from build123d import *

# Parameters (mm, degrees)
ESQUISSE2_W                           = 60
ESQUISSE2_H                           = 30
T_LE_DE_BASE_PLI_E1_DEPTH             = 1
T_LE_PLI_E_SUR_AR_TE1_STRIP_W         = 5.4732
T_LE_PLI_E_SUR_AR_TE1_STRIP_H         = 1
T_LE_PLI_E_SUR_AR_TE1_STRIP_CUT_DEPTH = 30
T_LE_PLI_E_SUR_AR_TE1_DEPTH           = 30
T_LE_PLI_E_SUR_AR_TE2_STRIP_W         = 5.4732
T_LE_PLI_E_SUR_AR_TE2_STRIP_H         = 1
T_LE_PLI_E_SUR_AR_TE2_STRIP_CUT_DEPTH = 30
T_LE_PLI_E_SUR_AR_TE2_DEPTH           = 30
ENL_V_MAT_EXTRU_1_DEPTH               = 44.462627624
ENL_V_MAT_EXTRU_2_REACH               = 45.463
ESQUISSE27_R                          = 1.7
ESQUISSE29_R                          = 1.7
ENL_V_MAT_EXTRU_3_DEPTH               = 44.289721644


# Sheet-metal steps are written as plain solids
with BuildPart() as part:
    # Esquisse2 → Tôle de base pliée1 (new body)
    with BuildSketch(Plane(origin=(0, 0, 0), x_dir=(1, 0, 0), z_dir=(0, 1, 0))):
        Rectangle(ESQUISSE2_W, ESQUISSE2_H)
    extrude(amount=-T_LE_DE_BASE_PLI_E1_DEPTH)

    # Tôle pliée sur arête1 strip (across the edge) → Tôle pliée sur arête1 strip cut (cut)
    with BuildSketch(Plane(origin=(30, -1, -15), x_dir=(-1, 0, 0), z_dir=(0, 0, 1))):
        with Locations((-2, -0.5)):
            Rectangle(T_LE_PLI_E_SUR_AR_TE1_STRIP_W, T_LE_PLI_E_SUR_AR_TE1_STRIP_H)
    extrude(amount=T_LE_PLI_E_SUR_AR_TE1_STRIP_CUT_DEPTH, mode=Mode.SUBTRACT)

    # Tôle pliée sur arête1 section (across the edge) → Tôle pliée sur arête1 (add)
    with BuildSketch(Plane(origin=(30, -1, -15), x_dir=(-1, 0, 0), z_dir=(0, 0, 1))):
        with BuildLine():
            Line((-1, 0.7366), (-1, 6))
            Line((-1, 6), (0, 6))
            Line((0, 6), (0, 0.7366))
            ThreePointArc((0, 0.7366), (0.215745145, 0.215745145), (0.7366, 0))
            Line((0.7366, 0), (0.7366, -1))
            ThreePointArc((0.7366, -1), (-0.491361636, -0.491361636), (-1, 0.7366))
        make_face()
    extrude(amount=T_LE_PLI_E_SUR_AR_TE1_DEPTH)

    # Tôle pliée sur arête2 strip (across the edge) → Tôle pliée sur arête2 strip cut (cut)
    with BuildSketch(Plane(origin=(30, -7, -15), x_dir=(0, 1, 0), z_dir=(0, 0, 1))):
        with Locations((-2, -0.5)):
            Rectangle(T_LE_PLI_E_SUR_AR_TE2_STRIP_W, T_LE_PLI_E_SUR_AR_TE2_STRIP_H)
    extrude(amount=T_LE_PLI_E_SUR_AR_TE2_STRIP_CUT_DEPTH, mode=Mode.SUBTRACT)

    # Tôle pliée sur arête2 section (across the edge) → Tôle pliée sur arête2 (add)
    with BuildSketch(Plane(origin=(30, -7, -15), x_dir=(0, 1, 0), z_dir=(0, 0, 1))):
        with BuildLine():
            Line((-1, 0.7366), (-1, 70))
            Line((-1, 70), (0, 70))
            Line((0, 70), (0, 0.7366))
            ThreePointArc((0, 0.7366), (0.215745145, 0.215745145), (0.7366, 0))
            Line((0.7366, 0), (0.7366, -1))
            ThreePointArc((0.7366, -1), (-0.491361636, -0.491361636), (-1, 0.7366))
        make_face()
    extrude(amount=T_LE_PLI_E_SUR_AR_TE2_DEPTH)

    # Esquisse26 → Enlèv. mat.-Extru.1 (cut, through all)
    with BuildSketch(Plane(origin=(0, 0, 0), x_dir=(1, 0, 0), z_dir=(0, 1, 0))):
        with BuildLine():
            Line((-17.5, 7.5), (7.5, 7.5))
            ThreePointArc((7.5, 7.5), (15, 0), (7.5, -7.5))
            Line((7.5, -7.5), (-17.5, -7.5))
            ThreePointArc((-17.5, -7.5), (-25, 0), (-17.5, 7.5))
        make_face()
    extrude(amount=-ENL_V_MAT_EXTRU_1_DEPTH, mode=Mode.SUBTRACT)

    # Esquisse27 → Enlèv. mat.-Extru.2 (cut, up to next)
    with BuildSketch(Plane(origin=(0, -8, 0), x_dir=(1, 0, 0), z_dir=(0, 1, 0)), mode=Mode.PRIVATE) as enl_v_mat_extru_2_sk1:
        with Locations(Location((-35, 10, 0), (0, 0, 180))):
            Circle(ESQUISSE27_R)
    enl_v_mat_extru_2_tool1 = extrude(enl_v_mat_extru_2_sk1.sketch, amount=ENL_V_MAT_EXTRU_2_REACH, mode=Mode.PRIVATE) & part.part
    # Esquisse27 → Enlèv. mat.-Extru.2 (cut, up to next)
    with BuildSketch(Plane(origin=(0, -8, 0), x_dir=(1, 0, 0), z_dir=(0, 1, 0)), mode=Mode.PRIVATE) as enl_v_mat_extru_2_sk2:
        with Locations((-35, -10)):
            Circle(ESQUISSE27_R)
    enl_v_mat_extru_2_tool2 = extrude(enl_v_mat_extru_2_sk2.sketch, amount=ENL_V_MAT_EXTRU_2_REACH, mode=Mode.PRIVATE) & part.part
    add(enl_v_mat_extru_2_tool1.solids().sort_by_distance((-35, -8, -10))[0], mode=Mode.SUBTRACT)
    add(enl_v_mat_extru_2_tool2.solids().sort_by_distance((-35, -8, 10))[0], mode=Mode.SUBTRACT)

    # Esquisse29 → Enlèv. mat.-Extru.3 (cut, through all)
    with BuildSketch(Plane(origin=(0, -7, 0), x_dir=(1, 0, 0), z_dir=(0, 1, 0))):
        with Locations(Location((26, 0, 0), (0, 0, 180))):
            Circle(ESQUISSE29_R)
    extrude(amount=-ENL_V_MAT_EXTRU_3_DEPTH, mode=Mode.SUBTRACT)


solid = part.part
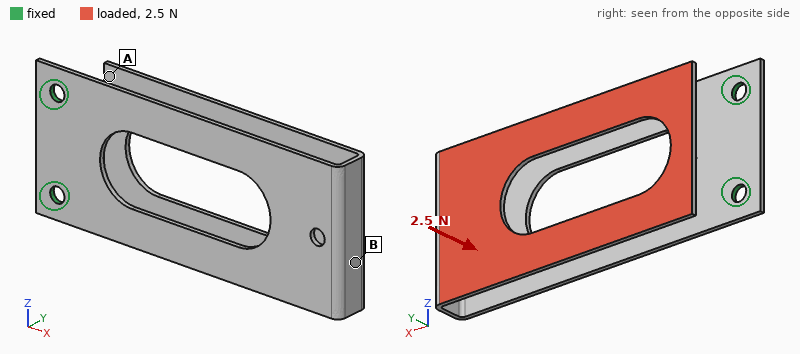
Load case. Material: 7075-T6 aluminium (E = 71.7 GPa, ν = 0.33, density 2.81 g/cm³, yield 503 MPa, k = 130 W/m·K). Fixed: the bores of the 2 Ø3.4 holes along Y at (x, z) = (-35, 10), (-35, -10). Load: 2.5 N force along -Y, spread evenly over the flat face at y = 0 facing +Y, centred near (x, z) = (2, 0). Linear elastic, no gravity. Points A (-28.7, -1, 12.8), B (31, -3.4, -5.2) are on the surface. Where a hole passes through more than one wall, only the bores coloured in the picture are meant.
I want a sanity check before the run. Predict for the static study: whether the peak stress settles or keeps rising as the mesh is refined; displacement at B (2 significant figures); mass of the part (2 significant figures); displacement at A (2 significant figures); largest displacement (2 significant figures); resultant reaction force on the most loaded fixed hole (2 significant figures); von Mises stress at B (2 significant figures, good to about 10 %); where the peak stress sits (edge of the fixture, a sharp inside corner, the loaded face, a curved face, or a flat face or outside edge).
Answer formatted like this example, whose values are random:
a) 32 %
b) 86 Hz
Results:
a) keeps rising
b) 0.62 mm
c) 8.4 g
d) 0.79 mm
e) 0.80 mm
f) 1.3 N
g) 13 MPa
h) edge of the fixture
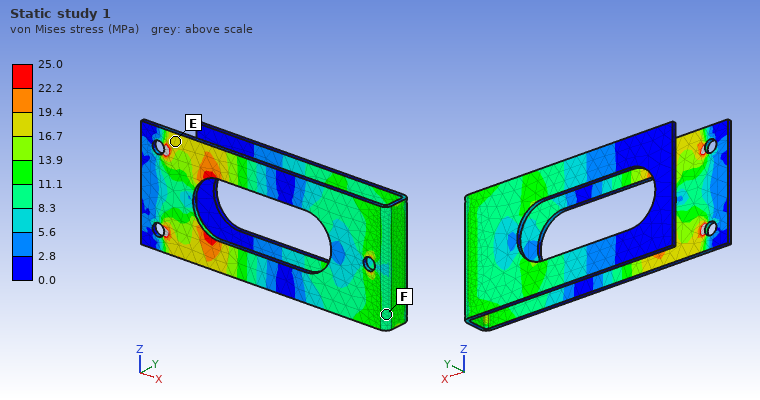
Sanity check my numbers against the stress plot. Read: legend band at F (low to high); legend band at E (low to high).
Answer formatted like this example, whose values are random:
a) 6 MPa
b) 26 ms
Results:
a) 8.3 to 11.1 MPa
b) 16.7 to 19.4 MPa
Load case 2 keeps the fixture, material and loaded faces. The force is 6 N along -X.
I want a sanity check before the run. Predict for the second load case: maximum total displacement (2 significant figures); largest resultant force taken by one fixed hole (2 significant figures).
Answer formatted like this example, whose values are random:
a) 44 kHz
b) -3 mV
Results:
a) 0.89 mm
b) 3.0 N
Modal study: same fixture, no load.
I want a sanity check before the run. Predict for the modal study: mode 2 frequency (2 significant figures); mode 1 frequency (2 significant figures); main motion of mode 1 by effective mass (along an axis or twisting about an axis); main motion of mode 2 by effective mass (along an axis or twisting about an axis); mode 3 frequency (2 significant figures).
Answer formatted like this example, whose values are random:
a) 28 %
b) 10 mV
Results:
a) 160 Hz
b) 110 Hz
c) along Y
d) along Y
e) 310 Hz
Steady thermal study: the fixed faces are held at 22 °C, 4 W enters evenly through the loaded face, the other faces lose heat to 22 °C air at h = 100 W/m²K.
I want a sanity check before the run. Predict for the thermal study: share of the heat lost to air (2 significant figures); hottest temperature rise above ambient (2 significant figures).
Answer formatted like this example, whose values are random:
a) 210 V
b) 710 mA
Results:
a) 97 %
b) 21 K
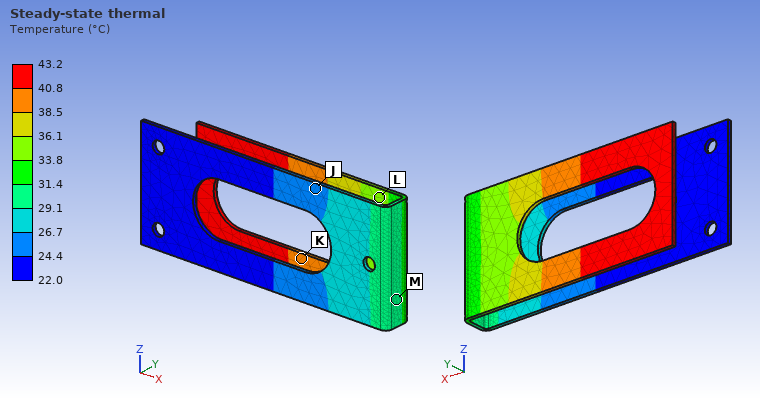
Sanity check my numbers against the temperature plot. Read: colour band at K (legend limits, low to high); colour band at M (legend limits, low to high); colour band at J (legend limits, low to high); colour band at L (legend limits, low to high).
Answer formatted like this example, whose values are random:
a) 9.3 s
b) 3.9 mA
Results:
a) 38.5 to 40.8 °C
b) 29.1 to 31.4 °C
c) 24.4 to 26.7 °C
d) 33.8 to 36.1 °C
